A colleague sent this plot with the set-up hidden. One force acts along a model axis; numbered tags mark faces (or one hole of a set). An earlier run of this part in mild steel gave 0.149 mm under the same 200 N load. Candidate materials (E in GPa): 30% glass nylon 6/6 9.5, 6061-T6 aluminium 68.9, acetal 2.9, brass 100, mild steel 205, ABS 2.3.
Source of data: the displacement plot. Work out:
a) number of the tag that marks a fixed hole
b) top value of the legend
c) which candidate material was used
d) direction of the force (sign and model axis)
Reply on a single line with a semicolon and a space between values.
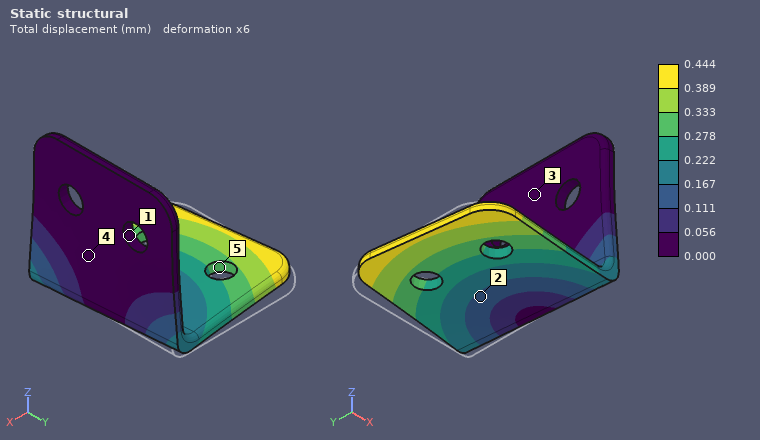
1; 0.444 mm; 6061-T6 aluminium; -Y
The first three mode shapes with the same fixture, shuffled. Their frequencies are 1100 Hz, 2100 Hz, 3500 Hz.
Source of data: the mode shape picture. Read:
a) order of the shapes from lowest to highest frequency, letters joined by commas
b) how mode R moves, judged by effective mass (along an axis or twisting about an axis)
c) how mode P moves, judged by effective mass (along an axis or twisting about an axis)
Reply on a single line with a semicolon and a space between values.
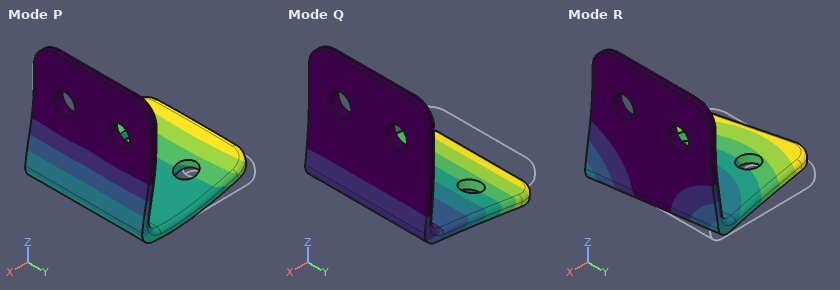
Q, R, P; along Y; along X
